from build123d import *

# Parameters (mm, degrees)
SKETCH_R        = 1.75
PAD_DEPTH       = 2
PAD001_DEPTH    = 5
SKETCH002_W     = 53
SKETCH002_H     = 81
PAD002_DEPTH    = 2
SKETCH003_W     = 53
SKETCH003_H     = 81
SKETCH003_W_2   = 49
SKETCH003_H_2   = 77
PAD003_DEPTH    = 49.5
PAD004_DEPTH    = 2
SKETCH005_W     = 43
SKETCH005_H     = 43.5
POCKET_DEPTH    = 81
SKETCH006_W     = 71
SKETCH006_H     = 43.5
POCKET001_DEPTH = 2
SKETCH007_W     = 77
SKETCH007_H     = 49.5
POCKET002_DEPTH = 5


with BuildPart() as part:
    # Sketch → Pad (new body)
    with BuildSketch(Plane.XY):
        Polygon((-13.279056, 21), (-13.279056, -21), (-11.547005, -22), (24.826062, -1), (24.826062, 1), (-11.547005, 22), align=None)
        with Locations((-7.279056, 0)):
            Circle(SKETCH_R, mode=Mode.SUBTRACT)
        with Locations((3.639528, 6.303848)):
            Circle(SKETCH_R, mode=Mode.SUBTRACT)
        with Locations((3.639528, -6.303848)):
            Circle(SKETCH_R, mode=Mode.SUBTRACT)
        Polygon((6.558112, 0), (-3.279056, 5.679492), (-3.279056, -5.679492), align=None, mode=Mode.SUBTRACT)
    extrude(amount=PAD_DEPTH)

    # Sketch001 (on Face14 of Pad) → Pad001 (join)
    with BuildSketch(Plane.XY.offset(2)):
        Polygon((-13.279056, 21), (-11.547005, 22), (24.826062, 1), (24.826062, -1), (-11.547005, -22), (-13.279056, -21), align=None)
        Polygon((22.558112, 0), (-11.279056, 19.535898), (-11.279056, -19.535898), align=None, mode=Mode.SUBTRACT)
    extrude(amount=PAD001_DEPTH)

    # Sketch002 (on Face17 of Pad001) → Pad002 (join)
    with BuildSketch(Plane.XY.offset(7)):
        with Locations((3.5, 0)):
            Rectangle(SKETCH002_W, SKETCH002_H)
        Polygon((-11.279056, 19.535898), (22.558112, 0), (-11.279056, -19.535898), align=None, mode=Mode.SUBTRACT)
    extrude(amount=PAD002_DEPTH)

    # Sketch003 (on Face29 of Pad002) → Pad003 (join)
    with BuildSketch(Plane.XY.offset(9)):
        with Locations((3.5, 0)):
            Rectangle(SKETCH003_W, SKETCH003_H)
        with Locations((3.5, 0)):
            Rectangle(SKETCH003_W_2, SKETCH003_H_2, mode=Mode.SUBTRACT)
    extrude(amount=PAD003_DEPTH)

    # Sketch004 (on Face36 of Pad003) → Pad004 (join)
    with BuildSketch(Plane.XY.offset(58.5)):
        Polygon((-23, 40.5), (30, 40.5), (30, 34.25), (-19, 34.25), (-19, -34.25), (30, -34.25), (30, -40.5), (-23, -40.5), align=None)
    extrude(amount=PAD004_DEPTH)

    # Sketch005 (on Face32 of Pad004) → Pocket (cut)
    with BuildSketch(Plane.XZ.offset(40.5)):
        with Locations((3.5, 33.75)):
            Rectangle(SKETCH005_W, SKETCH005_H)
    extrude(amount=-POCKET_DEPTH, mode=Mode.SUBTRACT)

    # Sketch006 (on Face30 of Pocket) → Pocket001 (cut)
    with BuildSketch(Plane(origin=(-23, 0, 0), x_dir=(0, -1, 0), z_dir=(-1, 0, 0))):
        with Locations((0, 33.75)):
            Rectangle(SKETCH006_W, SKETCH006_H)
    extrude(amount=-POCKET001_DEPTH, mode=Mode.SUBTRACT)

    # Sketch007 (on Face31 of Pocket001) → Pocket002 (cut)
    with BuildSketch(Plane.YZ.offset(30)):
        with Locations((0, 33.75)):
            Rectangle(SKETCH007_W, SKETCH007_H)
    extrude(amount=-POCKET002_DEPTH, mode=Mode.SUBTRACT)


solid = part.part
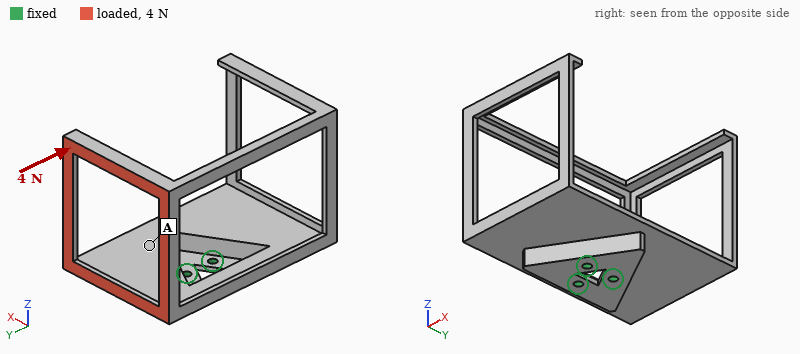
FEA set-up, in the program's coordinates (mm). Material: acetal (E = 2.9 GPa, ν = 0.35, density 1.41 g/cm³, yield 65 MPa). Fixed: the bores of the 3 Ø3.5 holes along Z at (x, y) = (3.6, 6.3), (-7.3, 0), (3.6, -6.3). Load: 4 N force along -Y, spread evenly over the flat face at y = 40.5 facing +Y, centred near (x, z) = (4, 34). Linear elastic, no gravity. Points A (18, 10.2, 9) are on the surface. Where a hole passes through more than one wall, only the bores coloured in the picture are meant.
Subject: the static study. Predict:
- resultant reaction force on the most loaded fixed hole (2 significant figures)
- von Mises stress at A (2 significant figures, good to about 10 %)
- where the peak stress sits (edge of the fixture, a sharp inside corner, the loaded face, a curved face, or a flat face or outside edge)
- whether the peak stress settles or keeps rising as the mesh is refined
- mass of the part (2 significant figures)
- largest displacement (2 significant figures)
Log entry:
5.9 N
0.42 MPa
a sharp inside corner
keeps rising
23 g
1.1 mm
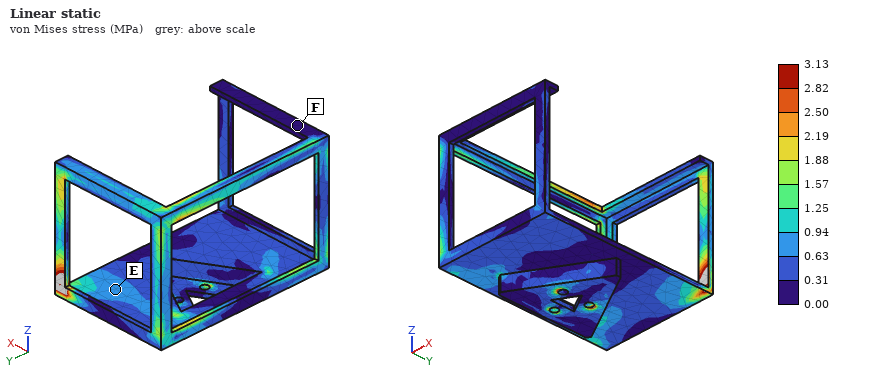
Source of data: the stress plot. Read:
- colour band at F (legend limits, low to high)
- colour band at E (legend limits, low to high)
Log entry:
0.00 to 0.31 MPa
0.63 to 0.94 MPa
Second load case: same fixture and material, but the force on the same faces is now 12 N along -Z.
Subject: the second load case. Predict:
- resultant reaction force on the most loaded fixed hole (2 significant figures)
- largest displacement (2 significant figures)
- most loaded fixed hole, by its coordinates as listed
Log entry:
31 N
1.4 mm
(3.6, 6.3)
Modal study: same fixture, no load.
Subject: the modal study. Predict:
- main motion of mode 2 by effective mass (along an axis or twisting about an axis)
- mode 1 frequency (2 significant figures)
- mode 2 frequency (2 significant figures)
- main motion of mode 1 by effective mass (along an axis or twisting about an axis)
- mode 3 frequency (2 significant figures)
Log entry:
along X
130 Hz
140 Hz
along Y
210 Hz
